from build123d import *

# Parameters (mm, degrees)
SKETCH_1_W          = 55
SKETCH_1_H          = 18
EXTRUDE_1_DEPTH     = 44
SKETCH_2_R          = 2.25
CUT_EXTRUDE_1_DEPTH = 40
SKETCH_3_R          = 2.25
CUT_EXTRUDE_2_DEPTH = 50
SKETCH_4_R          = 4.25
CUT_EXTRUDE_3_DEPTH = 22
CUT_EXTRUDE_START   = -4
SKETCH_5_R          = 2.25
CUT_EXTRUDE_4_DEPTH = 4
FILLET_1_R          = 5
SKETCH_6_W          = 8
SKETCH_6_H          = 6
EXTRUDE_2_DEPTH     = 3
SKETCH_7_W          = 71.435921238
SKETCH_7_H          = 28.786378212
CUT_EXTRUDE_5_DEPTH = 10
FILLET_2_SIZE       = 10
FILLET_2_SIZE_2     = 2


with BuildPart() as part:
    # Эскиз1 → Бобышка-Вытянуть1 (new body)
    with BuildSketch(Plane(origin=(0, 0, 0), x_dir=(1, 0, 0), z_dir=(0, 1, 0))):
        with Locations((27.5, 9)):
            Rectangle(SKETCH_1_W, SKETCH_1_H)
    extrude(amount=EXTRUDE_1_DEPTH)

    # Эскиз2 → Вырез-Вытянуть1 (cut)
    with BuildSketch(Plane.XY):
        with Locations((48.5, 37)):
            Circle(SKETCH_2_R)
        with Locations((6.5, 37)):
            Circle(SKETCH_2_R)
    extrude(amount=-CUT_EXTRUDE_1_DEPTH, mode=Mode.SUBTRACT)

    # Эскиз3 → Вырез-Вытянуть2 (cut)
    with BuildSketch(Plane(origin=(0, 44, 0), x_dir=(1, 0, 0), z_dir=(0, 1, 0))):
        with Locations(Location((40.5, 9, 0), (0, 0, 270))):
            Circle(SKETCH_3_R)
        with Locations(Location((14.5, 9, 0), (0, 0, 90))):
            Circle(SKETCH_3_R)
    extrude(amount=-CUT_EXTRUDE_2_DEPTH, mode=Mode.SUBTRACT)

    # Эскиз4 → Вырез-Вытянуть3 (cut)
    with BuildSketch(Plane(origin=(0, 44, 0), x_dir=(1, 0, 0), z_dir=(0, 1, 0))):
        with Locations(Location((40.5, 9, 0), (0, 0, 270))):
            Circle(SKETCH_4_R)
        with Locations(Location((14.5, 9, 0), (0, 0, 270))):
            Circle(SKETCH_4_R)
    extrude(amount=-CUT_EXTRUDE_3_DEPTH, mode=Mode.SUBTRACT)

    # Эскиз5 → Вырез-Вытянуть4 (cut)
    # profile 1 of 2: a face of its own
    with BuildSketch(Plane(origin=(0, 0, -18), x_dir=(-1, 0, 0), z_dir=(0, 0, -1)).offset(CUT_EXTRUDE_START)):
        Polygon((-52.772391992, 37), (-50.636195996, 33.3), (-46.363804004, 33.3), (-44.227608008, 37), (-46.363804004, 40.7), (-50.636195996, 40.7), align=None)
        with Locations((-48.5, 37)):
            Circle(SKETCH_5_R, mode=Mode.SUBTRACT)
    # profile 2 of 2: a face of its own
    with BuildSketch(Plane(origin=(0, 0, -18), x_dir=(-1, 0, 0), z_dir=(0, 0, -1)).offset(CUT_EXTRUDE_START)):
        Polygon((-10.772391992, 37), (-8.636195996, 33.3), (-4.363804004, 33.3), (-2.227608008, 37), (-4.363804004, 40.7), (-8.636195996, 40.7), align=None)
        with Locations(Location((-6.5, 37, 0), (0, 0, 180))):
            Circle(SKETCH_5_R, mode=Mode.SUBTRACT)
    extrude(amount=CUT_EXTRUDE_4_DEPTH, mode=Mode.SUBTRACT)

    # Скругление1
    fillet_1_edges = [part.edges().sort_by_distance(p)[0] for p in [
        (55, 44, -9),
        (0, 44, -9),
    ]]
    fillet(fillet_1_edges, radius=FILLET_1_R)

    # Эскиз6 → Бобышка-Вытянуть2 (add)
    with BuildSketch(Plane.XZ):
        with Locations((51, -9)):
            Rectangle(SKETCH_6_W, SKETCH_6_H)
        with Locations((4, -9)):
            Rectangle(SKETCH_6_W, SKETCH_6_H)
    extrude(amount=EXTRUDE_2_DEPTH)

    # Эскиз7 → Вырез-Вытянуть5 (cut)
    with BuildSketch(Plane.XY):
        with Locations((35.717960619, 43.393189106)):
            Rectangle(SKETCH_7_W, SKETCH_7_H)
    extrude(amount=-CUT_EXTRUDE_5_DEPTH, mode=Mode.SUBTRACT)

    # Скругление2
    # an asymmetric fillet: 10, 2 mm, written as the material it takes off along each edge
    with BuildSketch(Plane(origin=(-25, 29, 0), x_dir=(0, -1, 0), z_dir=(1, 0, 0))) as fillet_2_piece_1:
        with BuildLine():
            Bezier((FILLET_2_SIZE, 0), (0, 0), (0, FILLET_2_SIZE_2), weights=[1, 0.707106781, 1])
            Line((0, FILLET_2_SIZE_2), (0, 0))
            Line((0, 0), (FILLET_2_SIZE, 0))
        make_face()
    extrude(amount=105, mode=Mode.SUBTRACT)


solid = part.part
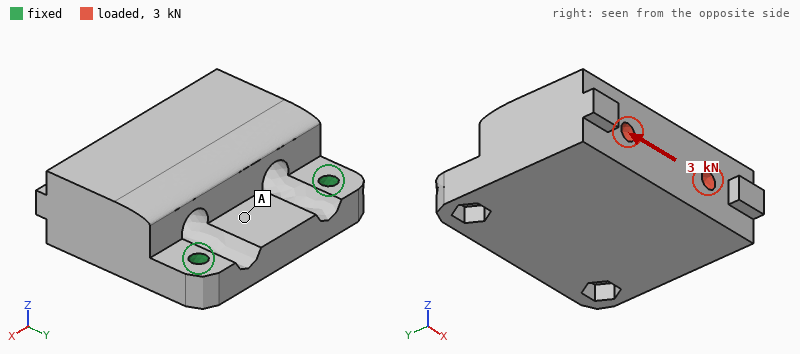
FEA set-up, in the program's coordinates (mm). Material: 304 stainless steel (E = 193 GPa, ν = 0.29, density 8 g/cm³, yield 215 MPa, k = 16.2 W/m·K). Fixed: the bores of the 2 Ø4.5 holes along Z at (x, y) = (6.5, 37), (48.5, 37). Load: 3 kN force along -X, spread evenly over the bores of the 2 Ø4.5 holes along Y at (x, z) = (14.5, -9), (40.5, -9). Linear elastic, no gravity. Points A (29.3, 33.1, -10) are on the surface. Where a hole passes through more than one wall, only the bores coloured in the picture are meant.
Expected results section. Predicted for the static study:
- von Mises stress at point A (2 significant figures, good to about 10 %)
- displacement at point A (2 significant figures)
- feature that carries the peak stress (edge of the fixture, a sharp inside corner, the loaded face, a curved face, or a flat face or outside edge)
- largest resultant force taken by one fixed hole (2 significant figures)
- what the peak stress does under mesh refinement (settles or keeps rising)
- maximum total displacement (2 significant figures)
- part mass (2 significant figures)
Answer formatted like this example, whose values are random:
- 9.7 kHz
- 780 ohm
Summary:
- 11 MPa
- 2.6 µm
- edge of the fixture
- 2.3 kN
- keeps rising
- 8.6 µm
- 260 g
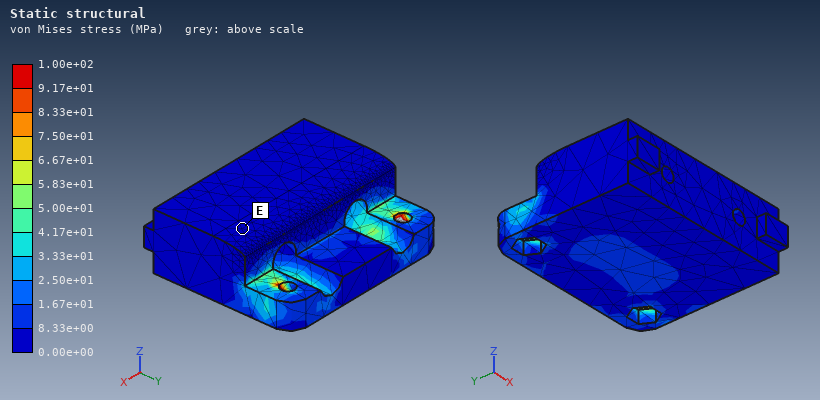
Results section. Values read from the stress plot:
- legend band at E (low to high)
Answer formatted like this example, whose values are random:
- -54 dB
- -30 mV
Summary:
- 0.00e+00 to 8.33e+00 MPa
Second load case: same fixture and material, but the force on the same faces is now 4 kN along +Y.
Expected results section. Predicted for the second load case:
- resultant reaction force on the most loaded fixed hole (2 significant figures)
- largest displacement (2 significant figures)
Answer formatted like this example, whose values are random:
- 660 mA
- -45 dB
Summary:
- 2.0 kN
- 45 µm
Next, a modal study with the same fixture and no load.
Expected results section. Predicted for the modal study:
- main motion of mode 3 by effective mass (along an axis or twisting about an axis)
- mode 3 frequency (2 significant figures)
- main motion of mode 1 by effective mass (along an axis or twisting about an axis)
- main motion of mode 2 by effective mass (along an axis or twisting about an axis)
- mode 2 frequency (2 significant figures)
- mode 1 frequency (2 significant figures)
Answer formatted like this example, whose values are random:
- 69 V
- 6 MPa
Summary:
- along X
- 8900 Hz
- along Z
- along X
- 6700 Hz
- 1700 Hz
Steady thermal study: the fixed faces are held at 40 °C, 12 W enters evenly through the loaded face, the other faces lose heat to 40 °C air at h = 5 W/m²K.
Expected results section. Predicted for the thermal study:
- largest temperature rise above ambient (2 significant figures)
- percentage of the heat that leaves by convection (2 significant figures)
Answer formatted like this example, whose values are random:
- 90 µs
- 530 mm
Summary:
- 51 K
- 13 %
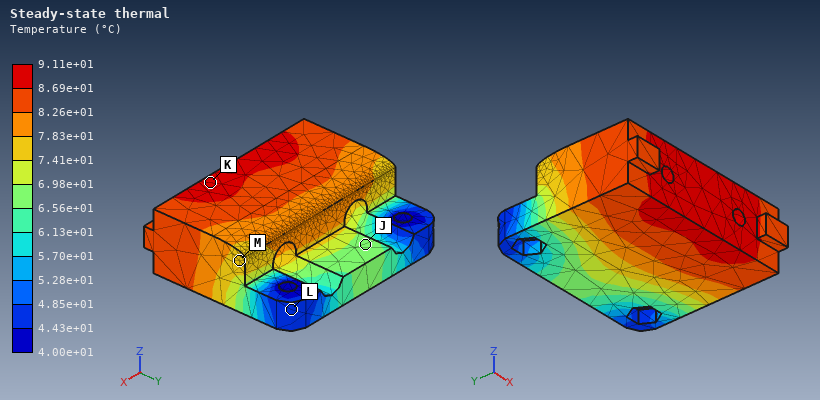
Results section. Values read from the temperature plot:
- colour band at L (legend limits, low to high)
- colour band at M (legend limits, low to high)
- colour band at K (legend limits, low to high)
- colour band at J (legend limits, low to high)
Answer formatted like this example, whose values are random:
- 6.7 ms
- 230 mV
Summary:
- 4.43e+01 to 4.85e+01 °C
- 7.41e+01 to 7.83e+01 °C
- 8.69e+01 to 9.11e+01 °C
- 6.56e+01 to 6.98e+01 °C
